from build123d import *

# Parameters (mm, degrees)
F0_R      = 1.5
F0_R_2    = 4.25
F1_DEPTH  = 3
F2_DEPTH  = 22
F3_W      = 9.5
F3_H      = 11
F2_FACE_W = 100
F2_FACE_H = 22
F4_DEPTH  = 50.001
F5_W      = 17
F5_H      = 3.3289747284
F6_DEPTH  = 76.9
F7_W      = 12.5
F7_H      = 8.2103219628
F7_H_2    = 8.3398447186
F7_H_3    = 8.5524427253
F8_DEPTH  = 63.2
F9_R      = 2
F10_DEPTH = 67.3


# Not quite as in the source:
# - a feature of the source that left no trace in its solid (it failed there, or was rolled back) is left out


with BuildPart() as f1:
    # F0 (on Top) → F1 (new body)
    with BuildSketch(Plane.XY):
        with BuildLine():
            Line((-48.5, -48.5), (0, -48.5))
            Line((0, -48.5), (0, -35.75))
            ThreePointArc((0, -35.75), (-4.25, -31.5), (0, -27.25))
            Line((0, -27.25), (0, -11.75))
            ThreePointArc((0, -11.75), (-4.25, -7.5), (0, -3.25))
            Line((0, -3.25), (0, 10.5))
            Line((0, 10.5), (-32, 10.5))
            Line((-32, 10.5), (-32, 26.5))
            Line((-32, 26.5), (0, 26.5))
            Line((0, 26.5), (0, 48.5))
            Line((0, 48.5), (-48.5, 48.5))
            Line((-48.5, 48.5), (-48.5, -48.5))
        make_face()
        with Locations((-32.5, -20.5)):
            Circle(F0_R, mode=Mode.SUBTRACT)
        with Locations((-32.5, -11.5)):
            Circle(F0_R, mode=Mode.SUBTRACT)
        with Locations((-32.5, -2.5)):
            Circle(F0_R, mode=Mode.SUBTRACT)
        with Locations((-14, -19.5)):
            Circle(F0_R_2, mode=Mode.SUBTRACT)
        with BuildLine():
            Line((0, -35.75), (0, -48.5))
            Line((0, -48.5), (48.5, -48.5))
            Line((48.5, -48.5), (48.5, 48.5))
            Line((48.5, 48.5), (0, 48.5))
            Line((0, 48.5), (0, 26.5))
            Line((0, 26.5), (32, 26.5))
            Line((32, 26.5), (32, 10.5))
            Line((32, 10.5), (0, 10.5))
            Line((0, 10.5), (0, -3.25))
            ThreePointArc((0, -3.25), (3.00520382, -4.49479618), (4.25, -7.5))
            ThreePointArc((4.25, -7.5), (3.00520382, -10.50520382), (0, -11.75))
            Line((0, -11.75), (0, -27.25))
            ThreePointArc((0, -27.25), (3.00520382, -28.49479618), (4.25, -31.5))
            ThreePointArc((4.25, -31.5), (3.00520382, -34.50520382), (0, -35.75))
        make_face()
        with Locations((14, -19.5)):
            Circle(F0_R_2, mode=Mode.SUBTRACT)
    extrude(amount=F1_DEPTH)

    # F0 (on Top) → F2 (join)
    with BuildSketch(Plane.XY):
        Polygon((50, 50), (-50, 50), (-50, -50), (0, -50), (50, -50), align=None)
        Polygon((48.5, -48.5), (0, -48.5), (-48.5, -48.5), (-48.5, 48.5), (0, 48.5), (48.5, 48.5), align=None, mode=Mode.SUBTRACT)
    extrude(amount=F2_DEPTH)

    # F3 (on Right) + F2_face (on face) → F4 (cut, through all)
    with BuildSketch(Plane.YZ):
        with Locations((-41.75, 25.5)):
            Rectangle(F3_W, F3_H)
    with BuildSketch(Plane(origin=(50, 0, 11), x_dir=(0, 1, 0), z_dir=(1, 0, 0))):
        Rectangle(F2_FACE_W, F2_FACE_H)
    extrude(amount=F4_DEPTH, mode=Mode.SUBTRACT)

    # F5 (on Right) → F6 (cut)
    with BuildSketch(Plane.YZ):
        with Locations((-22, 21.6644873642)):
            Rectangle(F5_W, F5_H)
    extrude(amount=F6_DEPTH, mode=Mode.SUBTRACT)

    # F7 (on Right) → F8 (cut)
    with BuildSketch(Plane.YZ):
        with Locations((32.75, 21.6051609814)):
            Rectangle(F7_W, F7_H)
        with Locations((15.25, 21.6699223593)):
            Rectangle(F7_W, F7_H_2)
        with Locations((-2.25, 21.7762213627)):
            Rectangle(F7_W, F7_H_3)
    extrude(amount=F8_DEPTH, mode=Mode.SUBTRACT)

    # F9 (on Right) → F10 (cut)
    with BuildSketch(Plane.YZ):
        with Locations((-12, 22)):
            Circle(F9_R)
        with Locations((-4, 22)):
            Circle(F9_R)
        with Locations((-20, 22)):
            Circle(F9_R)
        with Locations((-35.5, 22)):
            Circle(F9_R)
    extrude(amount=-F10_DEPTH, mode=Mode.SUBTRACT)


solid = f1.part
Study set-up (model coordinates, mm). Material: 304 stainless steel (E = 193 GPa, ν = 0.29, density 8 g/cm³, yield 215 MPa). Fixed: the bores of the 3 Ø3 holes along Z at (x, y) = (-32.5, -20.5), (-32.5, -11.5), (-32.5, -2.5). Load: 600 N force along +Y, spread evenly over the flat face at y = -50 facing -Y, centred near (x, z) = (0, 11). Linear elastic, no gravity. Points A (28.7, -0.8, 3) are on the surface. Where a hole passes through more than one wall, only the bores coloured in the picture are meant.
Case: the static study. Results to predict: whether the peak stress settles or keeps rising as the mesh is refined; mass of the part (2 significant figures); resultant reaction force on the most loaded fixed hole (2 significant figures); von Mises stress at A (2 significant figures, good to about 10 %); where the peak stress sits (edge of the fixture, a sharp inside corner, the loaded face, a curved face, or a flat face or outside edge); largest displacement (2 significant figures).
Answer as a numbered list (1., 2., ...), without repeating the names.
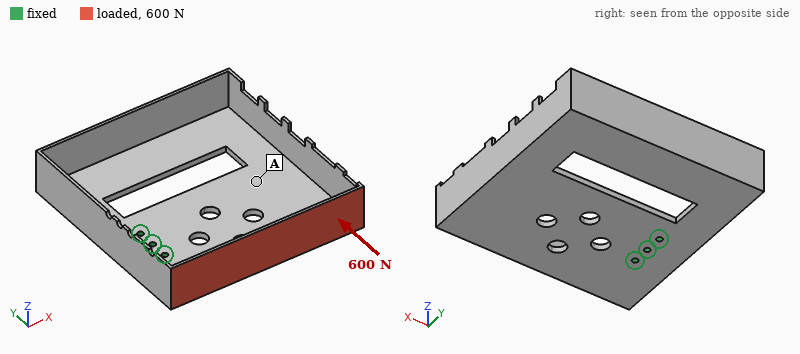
1. keeps rising
2. 300 g
3. 1.0 kN
4. 17 MPa
5. edge of the fixture
6. 0.20 mm
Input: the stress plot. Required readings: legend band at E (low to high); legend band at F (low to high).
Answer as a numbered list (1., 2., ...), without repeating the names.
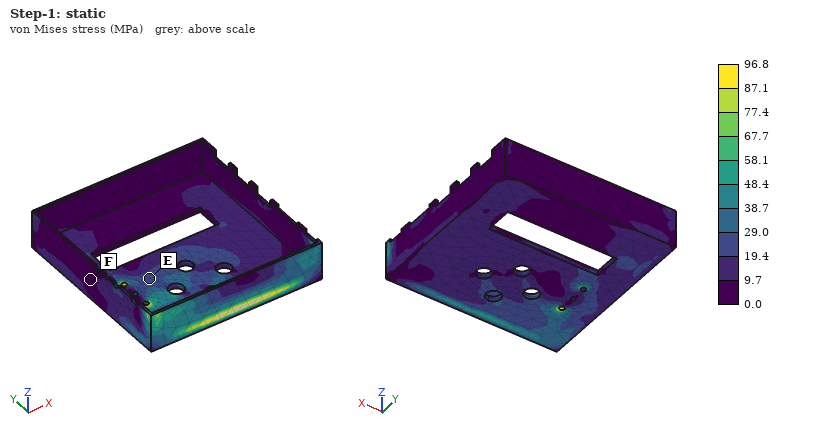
1. 19.4 to 29.0 MPa
2. 0.0 to 9.7 MPa
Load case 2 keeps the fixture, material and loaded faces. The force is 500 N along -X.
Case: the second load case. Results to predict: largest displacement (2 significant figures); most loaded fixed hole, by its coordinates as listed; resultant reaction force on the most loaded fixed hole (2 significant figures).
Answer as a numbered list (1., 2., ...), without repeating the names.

1. 0.27 mm
2. (-32.5, -20.5)
3. 1.2 kN
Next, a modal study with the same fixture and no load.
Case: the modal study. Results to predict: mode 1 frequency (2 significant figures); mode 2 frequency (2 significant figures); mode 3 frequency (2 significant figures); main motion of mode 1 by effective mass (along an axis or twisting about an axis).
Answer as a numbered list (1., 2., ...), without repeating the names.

1. 260 Hz
2. 450 Hz
3. 1000 Hz
4. along Z
